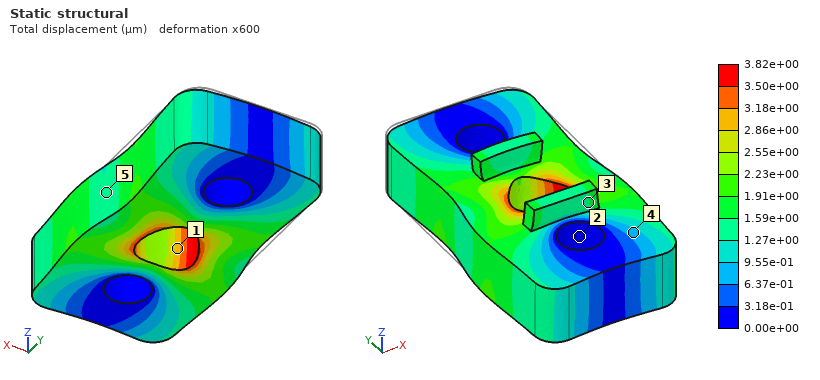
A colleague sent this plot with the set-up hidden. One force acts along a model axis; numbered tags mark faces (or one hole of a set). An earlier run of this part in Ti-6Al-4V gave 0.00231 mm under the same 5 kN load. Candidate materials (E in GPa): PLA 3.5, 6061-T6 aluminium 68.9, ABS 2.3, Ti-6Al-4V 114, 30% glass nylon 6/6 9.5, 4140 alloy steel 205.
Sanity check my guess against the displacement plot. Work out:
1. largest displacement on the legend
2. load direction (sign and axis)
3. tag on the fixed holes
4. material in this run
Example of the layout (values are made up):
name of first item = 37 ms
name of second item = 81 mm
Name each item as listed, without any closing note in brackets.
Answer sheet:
largest displacement on the legend = 3.82e+00 µm
load direction = -Y
tag on the fixed holes = 2
material in this run = 6061-T6 aluminium
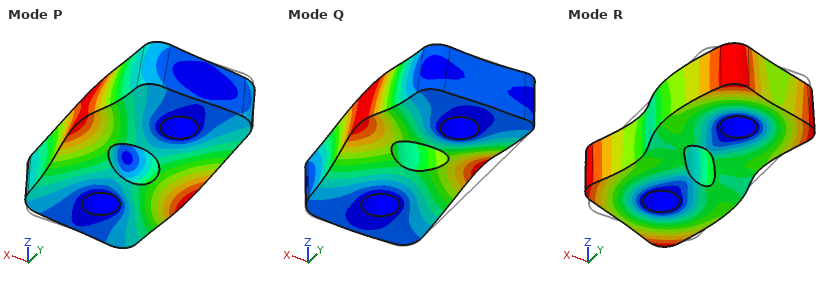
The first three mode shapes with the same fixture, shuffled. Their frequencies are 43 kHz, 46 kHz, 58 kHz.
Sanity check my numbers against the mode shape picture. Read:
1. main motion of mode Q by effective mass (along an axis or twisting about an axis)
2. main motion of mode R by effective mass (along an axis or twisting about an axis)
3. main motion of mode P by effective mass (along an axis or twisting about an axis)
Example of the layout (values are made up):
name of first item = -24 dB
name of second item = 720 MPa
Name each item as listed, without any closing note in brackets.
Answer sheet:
main motion of mode Q by effective mass = along Z
main motion of mode R by effective mass = twisting about Z
main motion of mode P by effective mass = twisting about Y
